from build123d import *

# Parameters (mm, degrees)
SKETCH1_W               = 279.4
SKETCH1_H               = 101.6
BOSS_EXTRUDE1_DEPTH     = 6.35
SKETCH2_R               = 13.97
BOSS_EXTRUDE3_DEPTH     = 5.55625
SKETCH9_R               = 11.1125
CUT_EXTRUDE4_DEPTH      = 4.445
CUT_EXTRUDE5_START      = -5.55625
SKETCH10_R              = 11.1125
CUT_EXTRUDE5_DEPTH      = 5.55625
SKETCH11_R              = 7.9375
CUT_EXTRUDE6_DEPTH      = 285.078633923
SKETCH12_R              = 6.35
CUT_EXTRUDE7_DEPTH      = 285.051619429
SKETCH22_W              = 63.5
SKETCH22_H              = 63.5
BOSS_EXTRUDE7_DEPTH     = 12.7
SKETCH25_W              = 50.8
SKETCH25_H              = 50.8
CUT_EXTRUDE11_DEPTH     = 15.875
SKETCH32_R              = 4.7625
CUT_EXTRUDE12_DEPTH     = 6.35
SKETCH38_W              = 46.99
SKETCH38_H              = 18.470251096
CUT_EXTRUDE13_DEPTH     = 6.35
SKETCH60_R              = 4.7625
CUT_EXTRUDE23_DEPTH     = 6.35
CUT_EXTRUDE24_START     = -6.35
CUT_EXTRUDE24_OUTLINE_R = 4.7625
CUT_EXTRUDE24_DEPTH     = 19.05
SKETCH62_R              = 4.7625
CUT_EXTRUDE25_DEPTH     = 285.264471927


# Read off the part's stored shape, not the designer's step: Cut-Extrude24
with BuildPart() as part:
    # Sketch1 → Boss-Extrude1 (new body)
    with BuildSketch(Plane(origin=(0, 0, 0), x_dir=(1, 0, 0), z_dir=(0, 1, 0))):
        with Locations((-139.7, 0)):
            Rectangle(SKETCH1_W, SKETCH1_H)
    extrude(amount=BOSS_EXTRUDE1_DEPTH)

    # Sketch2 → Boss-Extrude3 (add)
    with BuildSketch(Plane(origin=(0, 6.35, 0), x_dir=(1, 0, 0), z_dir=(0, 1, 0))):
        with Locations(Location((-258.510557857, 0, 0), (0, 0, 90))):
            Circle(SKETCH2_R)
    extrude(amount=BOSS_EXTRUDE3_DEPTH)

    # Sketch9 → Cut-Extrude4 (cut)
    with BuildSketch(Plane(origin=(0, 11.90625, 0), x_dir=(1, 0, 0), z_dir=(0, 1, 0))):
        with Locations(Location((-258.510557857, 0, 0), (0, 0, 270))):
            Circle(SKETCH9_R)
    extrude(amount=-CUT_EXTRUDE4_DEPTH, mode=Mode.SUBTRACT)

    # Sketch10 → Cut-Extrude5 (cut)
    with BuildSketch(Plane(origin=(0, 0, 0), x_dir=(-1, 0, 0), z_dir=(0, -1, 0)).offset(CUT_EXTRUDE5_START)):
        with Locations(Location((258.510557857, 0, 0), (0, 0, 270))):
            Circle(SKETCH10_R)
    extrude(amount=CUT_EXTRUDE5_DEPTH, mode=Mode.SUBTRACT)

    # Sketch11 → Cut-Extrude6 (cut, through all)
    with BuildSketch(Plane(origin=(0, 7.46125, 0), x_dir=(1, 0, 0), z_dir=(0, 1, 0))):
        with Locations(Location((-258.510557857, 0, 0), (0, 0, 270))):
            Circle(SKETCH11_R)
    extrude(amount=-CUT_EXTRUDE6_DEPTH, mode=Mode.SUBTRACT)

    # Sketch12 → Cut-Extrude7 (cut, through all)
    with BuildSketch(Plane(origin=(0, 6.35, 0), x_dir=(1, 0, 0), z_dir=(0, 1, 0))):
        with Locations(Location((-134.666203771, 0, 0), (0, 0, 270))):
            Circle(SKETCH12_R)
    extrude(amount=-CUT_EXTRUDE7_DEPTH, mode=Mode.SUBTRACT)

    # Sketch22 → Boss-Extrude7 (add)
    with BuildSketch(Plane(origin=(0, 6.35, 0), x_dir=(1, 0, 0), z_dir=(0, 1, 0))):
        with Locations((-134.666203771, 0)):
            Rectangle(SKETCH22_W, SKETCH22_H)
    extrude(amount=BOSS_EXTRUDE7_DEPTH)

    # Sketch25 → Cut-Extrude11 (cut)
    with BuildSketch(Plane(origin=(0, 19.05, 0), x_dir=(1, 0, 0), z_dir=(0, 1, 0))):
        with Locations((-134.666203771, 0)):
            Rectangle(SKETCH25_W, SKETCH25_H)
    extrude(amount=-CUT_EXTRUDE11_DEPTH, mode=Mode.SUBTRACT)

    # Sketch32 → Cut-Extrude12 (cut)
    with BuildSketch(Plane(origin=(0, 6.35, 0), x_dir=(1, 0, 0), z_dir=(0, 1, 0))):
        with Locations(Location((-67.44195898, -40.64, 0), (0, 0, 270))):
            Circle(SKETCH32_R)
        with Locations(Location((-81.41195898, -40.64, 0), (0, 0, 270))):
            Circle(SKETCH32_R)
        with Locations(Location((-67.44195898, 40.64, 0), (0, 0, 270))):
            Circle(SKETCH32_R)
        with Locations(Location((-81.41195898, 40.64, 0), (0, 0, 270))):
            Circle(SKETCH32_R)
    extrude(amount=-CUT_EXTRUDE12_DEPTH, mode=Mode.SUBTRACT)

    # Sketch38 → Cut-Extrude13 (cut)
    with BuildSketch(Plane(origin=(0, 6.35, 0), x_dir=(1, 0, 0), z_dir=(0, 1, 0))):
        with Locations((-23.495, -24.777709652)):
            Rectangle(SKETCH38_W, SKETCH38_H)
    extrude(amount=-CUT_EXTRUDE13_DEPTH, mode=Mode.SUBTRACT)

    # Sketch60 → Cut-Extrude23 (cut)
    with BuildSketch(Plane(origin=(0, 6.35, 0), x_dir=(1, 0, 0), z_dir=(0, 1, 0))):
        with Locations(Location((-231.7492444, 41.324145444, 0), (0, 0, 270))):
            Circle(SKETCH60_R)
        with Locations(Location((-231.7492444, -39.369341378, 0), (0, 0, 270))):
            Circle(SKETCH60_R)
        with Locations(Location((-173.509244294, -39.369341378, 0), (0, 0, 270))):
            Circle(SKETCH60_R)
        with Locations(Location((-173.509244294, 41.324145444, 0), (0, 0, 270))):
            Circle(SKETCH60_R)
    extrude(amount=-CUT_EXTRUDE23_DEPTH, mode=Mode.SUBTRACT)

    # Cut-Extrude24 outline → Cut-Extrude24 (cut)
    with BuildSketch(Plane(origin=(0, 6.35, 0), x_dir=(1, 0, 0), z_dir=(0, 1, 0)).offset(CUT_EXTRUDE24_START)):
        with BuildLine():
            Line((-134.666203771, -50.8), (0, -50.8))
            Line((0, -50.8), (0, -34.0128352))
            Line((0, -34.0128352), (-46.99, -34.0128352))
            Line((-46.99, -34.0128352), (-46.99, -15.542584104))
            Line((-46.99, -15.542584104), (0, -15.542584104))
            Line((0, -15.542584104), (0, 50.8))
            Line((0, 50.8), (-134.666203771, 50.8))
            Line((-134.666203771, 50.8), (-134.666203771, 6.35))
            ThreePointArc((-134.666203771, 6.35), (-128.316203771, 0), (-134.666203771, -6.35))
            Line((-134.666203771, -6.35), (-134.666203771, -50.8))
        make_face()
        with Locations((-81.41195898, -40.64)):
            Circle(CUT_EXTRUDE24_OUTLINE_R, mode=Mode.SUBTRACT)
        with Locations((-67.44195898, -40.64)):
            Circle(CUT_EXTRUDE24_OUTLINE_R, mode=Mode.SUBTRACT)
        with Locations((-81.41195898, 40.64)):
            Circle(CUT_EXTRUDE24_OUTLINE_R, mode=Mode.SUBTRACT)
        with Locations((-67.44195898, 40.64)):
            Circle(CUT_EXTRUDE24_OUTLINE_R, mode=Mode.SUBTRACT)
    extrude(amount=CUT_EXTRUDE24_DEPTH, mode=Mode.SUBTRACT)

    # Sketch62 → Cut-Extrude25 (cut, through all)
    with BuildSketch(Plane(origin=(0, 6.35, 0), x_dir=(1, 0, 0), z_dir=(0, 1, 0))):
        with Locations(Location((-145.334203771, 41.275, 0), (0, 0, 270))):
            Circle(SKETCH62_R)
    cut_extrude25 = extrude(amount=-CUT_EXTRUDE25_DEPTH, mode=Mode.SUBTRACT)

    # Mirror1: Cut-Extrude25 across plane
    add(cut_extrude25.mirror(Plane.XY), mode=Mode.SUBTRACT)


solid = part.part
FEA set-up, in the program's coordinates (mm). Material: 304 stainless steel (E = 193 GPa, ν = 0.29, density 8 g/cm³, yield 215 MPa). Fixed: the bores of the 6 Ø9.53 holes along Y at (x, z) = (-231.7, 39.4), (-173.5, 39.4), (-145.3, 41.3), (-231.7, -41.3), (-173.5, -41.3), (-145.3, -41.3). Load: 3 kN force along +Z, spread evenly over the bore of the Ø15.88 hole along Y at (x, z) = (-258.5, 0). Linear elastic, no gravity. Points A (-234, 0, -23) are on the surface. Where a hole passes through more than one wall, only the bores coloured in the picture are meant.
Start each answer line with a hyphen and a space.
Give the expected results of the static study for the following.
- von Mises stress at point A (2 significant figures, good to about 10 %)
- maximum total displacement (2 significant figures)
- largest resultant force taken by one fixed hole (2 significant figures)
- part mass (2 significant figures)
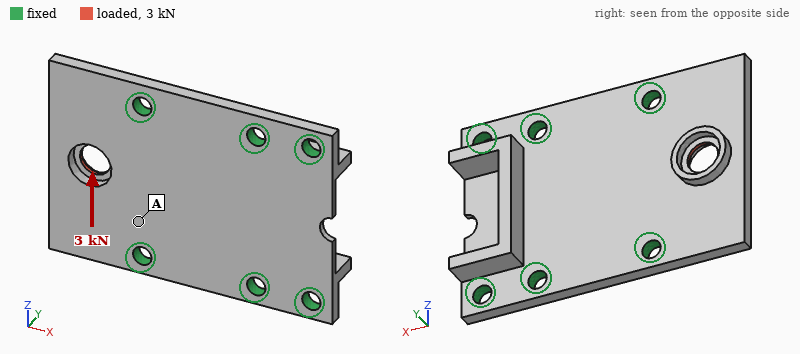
- 5.7 MPa
- 7.4 µm
- 1.7 kN
- 760 g
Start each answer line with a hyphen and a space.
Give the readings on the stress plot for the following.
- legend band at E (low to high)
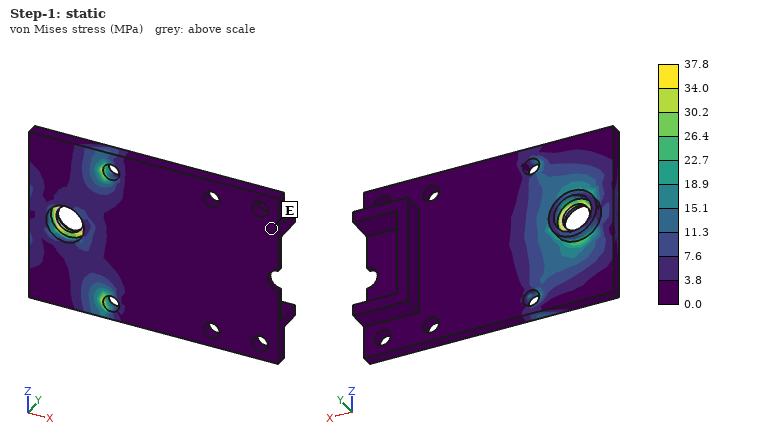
- 0.0 to 3.8 MPa
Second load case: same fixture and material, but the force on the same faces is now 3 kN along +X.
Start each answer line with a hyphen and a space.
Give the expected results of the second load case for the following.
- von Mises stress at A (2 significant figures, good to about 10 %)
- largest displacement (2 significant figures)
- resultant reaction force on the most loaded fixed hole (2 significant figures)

- 6.1 MPa
- 28 µm
- 1.1 kN
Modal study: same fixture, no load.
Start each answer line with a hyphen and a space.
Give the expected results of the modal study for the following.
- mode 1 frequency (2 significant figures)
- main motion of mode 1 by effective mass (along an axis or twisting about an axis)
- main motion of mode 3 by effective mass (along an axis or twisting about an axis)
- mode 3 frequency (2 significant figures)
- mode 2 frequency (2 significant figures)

- 2000 Hz
- along Y
- along Y
- 4900 Hz
- 3400 Hz
